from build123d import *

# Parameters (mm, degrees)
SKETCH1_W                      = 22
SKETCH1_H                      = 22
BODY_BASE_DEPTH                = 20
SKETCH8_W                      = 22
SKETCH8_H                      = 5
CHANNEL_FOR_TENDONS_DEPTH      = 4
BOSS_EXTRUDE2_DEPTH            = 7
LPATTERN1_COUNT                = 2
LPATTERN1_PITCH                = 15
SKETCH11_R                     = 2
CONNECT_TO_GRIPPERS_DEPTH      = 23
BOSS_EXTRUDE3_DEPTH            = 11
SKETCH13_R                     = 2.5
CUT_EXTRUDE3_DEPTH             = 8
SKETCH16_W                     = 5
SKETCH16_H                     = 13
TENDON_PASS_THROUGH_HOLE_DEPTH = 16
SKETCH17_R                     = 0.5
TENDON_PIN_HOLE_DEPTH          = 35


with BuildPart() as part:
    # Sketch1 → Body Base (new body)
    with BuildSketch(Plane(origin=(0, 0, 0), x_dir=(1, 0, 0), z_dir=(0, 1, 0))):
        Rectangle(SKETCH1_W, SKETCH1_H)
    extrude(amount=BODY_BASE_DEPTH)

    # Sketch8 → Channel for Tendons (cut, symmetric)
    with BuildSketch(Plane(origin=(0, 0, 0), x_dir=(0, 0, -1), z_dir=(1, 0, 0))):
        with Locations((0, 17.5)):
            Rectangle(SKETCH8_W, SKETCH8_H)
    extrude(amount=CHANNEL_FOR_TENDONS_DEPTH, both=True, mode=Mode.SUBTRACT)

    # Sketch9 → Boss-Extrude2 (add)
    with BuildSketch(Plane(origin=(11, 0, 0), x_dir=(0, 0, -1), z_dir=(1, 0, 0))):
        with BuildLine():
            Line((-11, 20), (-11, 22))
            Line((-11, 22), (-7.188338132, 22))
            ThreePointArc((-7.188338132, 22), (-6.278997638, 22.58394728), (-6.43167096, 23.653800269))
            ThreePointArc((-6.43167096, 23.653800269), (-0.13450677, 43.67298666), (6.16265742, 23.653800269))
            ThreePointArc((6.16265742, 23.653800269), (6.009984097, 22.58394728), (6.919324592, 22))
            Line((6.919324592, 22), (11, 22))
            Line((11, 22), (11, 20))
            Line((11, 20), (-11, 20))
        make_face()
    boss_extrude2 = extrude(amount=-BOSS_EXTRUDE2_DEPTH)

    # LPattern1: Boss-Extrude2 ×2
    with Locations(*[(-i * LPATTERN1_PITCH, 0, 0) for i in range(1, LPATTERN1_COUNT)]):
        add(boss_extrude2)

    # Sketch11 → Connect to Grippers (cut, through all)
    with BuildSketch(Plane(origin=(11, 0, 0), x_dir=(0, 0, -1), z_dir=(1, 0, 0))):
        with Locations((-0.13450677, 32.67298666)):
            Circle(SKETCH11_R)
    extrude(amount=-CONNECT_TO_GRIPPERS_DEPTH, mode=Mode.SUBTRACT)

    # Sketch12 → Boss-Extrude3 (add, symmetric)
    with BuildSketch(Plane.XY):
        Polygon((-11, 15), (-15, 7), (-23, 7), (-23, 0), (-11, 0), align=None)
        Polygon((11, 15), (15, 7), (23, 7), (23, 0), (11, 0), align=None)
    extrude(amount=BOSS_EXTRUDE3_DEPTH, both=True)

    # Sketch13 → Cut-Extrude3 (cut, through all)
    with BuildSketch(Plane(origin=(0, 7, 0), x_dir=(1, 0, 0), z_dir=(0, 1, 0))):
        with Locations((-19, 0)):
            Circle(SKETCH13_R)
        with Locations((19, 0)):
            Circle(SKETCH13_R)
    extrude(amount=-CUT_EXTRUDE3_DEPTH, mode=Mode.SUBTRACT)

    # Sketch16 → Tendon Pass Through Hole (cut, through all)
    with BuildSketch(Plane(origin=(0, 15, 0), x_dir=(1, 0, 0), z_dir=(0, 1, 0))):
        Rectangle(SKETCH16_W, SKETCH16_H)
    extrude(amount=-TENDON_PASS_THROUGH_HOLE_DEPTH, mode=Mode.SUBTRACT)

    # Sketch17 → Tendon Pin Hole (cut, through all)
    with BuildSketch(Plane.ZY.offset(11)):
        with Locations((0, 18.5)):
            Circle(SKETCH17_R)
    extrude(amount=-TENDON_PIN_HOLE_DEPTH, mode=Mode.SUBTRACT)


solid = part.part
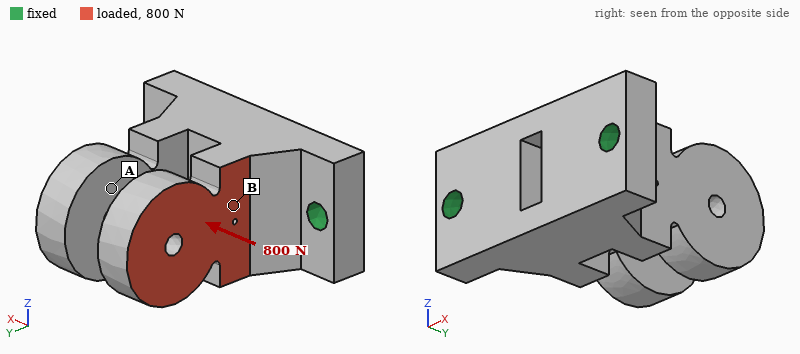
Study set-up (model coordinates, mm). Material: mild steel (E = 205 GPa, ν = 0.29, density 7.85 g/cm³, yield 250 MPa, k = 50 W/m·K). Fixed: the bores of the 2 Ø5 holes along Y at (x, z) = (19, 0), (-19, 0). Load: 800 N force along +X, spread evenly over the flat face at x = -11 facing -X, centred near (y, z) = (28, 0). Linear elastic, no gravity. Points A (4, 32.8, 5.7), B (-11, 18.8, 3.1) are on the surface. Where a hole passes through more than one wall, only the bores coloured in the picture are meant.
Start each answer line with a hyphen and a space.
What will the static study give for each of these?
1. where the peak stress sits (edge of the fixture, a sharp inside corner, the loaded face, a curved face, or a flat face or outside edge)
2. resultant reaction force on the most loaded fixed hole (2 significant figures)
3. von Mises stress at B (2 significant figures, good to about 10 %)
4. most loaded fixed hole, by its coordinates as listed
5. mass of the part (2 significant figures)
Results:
- a curved face
- 840 N
- 62 MPa
- (19, 0)
- 140 g
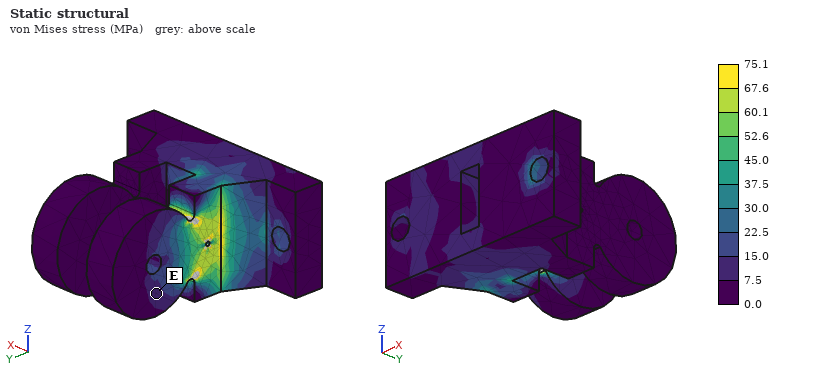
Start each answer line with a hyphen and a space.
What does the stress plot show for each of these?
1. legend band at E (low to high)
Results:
- 7.5 to 15.0 MPa
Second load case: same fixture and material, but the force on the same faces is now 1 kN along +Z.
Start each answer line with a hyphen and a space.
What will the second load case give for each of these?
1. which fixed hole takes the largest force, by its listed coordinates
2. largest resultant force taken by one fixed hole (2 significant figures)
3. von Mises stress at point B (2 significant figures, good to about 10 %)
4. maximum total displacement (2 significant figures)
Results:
- (-19, 0)
- 790 N
- 21 MPa
- 35 µm
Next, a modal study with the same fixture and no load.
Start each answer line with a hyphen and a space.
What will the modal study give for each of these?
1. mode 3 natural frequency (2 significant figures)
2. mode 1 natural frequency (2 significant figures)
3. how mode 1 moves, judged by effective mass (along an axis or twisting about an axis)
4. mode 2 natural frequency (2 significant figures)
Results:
- 5500 Hz
- 4700 Hz
- along Z
- 5300 Hz
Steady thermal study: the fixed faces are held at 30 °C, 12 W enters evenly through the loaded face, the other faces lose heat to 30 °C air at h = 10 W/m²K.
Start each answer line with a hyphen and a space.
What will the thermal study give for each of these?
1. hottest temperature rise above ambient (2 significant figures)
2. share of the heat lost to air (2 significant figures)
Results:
- 45 K
- 6.1 %
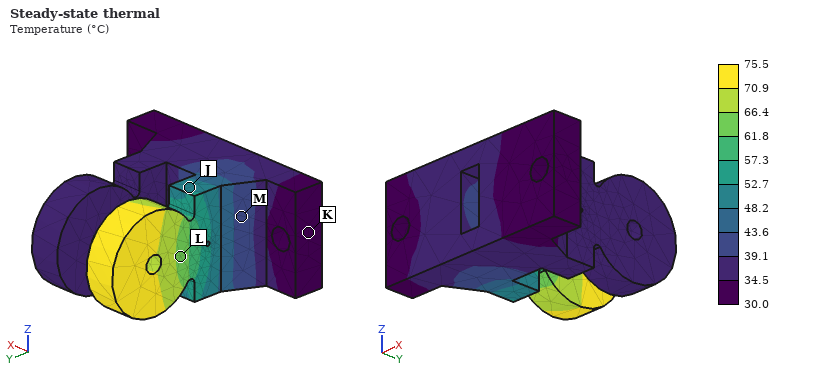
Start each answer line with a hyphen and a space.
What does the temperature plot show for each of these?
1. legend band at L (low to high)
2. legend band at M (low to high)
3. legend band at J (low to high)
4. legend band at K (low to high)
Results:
- 61.8 to 66.4 °C
- 39.1 to 43.6 °C
- 48.2 to 52.7 °C
- 30.0 to 34.5 °C
